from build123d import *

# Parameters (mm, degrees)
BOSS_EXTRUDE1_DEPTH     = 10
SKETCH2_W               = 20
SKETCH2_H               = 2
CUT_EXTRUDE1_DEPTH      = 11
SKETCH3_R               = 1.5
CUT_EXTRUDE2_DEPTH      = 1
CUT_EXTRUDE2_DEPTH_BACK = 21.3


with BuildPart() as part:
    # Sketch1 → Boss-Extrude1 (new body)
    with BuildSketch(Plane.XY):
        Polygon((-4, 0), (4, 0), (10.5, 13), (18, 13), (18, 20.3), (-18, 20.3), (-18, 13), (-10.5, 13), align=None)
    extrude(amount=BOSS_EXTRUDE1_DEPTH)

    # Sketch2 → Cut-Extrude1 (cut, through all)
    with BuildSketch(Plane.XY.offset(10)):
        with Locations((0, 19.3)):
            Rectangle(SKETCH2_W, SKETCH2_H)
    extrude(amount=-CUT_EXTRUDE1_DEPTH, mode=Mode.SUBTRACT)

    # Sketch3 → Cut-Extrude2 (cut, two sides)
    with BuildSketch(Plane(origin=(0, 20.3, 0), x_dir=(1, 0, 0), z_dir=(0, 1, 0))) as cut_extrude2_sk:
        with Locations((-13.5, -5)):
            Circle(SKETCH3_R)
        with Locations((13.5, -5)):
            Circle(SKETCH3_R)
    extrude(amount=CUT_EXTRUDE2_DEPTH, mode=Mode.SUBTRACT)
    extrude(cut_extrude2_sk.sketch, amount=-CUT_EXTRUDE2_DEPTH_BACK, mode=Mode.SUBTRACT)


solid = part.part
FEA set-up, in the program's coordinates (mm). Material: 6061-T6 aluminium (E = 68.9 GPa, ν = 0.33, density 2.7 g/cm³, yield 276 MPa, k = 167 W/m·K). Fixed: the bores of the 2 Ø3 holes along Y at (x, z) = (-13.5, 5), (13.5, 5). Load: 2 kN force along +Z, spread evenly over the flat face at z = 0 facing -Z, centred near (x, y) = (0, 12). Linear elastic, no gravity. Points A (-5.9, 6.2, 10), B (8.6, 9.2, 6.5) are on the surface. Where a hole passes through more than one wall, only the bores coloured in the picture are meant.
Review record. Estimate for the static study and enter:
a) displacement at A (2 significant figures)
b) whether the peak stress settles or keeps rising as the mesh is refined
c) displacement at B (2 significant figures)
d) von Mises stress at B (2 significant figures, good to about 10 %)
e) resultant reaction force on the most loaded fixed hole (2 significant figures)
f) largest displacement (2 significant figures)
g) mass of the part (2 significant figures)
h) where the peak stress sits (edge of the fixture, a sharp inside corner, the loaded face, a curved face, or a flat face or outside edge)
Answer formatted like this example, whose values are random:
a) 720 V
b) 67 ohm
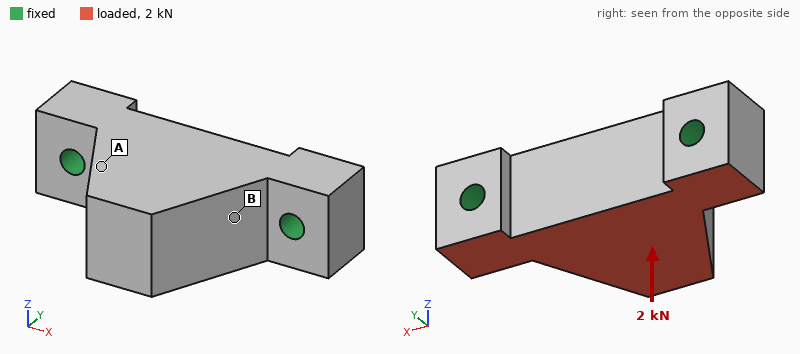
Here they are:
a) 24 µm
b) keeps rising
c) 16 µm
d) 31 MPa
e) 1.0 kN
f) 37 µm
g) 11 g
h) edge of the fixture
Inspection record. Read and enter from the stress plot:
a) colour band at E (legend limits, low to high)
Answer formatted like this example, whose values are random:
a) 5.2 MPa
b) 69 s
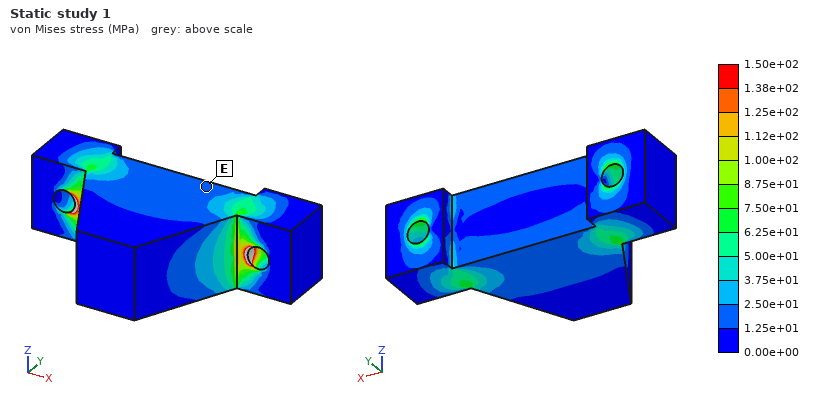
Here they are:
a) 1.25e+01 to 2.50e+01 MPa
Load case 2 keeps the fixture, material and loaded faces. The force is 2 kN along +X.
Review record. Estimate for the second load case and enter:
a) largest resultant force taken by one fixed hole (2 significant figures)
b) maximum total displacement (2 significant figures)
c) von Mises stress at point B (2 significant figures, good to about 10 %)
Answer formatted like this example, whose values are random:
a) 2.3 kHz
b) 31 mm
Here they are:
a) 1.1 kN
b) 7.0 µm
c) 11 MPa
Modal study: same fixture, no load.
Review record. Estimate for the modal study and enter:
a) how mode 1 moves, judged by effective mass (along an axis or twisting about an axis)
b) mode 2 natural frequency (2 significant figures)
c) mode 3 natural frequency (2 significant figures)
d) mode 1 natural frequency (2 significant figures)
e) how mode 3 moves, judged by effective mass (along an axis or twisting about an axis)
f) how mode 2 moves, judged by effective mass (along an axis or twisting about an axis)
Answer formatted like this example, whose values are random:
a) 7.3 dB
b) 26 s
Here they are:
a) along Z
b) 33 kHz
c) 38 kHz
d) 14 kHz
e) along X
f) along Y
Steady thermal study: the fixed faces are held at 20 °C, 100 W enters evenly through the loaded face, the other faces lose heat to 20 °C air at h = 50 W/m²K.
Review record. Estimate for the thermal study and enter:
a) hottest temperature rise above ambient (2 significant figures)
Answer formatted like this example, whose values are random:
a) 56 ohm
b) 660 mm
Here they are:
a) 40 K
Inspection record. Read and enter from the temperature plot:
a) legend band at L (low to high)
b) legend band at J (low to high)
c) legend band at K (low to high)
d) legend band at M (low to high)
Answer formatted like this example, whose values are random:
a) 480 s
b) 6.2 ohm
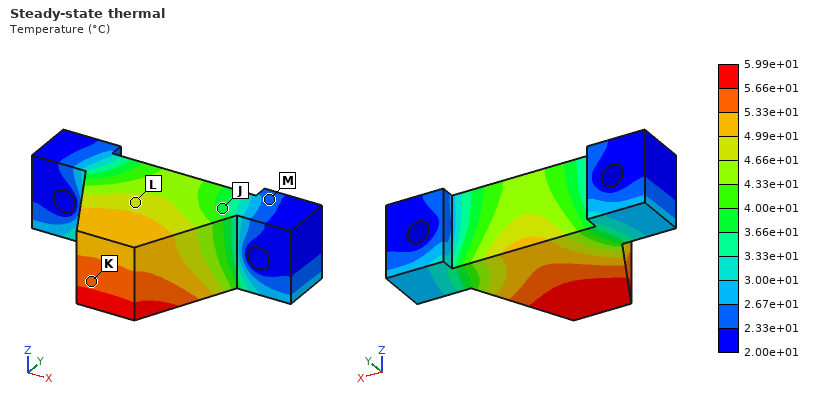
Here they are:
a) 4.66e+01 to 4.99e+01 °C
b) 3.66e+01 to 4.00e+01 °C
c) 5.33e+01 to 5.66e+01 °C
d) 2.33e+01 to 2.67e+01 °C
